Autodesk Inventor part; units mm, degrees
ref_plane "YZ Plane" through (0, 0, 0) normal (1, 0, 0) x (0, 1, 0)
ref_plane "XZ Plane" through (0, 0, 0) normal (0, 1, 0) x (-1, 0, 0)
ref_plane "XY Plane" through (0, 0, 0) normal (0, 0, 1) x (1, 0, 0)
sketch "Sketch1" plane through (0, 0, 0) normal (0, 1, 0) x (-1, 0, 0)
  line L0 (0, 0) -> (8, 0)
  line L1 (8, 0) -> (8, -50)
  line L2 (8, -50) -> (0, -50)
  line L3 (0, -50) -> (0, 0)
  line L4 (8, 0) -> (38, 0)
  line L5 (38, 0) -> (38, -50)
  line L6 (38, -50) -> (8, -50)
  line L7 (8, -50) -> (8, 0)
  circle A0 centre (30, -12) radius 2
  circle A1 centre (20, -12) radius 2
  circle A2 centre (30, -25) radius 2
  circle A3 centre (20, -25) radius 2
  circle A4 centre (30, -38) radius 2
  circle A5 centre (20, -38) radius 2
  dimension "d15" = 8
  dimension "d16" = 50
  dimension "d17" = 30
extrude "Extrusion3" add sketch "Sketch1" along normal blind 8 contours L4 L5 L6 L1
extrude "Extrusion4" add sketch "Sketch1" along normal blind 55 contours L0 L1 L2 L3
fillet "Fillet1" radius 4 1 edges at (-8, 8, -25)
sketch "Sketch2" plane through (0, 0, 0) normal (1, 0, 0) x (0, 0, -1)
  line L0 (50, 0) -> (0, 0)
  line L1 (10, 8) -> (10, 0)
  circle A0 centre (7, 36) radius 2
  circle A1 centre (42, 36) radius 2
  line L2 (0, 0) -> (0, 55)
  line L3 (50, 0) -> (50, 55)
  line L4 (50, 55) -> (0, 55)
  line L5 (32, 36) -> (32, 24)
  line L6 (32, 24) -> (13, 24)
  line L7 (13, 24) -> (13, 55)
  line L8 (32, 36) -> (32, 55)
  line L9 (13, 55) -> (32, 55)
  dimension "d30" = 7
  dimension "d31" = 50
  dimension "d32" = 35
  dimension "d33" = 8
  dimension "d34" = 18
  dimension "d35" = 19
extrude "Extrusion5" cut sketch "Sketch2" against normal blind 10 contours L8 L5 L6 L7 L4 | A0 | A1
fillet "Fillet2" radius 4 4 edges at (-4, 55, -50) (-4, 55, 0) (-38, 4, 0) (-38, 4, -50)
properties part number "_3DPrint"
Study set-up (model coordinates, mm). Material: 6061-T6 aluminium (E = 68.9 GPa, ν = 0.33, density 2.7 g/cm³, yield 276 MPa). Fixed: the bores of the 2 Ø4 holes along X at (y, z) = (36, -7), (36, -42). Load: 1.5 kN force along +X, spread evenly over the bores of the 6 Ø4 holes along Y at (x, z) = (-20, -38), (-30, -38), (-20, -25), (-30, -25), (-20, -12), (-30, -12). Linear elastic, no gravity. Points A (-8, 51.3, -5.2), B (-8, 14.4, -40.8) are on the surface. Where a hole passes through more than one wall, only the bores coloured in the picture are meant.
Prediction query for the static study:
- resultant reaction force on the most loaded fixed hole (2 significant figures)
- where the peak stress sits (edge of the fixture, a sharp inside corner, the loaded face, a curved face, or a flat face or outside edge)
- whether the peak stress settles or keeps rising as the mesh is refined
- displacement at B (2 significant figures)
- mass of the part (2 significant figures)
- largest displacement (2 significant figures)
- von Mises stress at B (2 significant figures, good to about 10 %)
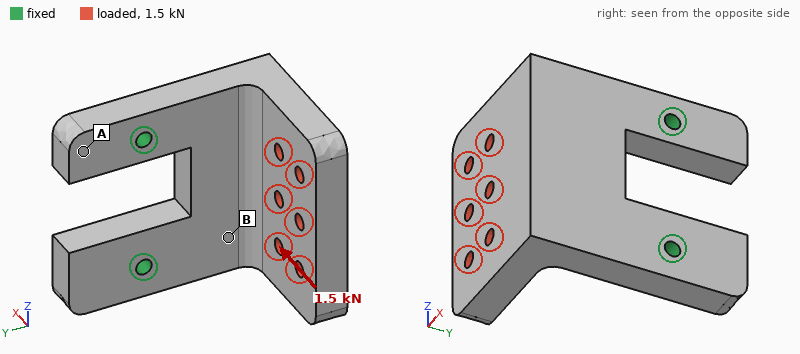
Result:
790 N
edge of the fixture
keeps rising
0.11 mm
77 g
0.35 mm
37 MPa
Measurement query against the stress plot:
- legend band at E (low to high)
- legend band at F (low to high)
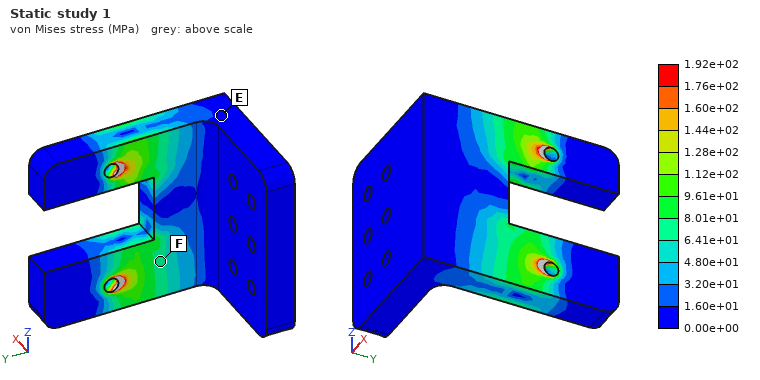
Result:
0.00e+00 to 1.60e+01 MPa
6.41e+01 to 8.01e+01 MPa
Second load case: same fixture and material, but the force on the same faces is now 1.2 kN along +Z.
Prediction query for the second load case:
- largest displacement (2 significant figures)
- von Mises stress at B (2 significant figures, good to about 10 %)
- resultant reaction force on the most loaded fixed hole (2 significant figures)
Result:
99 µm
31 MPa
1.2 kN
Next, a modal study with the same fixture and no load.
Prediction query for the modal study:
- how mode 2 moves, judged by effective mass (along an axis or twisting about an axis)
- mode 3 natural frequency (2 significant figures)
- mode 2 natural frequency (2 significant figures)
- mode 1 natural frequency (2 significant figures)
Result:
along Z
5600 Hz
3400 Hz
1700 Hz
